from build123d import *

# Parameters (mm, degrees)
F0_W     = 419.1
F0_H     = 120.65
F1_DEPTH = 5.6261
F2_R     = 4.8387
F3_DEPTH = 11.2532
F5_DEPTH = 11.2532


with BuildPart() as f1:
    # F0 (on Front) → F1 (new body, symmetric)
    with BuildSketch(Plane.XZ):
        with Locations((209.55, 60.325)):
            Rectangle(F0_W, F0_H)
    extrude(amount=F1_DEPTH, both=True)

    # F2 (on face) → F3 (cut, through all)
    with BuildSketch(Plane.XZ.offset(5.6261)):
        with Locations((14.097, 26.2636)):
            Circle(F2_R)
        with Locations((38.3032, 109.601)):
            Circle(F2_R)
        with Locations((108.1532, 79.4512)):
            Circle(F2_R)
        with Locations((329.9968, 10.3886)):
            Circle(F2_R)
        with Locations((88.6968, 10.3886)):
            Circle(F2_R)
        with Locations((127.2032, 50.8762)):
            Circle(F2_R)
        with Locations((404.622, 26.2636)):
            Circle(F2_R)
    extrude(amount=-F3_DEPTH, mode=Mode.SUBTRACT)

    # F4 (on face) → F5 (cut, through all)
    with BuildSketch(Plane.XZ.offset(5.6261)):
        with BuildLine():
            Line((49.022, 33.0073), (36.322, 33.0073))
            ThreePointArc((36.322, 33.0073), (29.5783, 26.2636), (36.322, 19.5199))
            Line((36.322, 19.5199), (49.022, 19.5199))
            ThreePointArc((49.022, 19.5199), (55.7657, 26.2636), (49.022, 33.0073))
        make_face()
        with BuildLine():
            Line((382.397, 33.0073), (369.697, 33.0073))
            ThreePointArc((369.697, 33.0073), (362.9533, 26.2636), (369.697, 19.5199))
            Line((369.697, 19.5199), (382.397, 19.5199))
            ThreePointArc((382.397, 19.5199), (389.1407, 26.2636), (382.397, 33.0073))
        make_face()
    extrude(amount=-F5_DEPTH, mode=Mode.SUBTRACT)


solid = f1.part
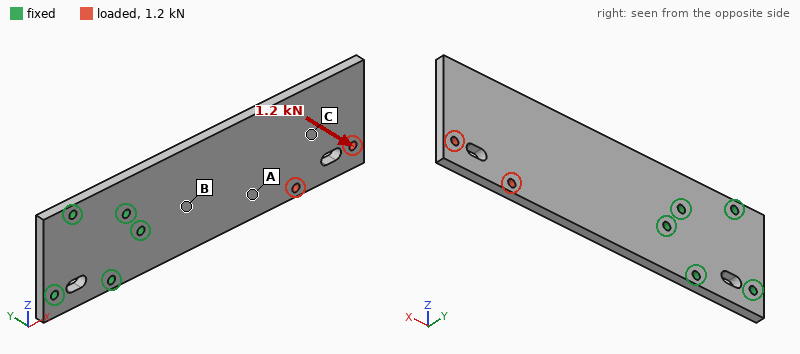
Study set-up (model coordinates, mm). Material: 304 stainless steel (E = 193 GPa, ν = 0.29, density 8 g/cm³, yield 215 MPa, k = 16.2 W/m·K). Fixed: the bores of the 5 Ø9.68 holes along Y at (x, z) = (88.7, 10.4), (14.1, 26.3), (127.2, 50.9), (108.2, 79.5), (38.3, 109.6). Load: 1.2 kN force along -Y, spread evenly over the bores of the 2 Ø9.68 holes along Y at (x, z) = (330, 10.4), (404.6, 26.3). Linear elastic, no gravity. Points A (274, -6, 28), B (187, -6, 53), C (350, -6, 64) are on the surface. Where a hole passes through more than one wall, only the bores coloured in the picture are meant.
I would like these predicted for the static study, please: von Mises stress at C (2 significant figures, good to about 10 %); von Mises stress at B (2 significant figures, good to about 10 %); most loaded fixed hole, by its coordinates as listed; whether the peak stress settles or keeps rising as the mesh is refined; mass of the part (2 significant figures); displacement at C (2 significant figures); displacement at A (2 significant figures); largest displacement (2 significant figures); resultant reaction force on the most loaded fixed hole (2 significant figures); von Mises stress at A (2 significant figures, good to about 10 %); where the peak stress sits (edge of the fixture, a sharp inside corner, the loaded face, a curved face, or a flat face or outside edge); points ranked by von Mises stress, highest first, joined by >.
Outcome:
17 MPa
78 MPa
(127.2, 50.9)
keeps rising
4.4 kg
1.8 mm
0.99 mm
2.9 mm
5.9 kN
48 MPa
edge of the fixture
B > A > C
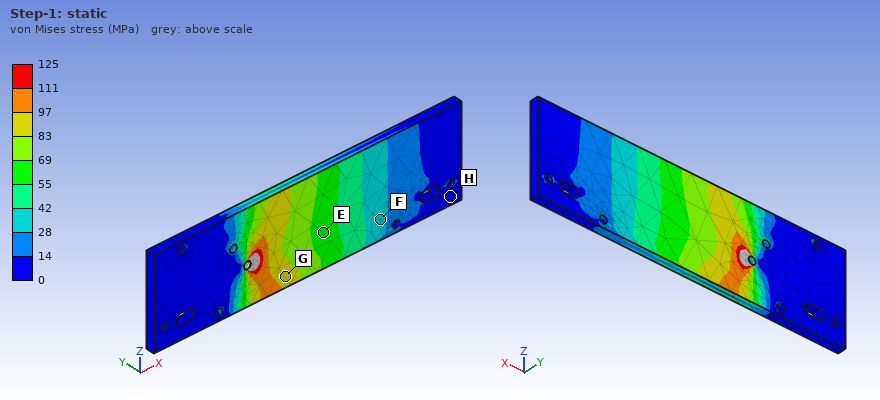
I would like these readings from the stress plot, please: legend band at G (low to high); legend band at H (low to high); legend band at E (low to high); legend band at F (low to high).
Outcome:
83 to 97 MPa
0 to 14 MPa
55 to 69 MPa
28 to 42 MPa
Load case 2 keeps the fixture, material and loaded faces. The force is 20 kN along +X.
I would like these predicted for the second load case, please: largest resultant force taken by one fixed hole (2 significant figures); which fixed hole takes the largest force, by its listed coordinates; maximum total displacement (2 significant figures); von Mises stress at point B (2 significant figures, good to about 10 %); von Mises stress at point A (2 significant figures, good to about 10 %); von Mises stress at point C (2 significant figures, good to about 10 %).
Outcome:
12 kN
(127.2, 50.9)
0.15 mm
20 MPa
31 MPa
11 MPa
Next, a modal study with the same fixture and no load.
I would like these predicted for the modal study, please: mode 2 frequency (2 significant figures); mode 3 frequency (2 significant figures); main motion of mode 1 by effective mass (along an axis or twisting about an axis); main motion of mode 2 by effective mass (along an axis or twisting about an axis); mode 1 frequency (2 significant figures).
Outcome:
490 Hz
630 Hz
along Y
twisting about X
100 Hz
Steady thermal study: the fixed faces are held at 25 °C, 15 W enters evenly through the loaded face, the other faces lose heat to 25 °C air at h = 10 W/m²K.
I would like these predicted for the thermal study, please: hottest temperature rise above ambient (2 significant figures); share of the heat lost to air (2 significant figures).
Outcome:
59 K
92 %
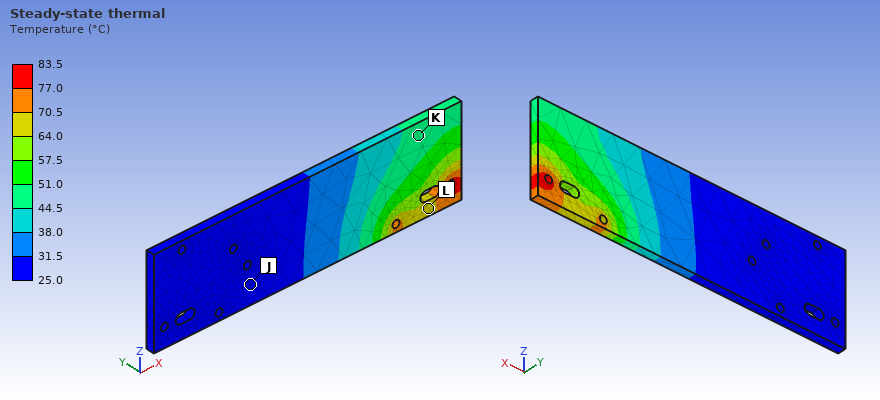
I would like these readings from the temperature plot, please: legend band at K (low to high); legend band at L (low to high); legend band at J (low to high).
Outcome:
44.5 to 51.0 °C
64.0 to 70.5 °C
25.0 to 31.5 °C
